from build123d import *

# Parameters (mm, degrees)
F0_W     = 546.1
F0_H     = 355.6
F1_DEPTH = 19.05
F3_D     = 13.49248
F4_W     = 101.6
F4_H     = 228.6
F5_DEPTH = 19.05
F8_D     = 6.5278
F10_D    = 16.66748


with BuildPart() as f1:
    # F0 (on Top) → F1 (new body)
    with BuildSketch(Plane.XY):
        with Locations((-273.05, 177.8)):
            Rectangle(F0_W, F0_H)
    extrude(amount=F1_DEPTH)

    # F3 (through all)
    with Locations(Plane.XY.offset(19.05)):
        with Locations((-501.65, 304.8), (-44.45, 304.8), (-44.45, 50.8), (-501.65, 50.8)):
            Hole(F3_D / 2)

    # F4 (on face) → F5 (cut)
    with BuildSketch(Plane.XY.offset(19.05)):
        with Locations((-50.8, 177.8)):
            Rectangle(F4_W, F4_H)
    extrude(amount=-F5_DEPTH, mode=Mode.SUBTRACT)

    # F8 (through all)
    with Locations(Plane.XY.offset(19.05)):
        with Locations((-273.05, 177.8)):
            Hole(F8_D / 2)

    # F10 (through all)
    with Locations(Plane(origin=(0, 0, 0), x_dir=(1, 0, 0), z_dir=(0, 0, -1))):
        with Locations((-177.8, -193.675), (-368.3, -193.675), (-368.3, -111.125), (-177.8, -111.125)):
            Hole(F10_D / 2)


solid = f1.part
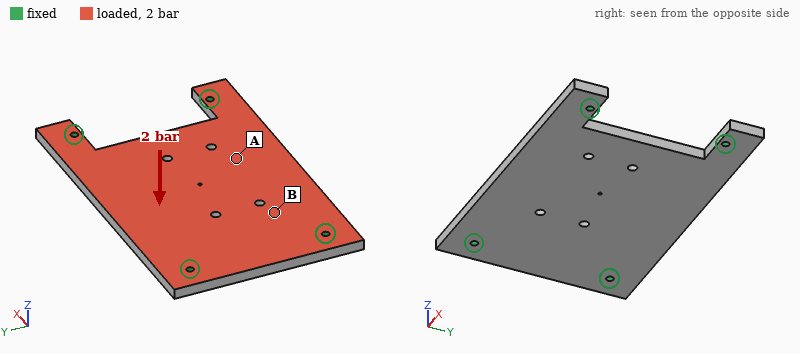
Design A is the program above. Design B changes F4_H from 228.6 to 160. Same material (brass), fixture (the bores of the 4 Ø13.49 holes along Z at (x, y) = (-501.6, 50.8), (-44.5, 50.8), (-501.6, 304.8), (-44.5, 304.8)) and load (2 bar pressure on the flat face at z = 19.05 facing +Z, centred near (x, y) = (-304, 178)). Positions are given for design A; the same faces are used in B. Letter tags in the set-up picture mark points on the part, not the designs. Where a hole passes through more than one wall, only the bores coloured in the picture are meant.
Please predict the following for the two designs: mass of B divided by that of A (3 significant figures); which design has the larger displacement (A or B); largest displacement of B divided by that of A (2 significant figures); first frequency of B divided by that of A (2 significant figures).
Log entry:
1.04
A
0.90
1.1
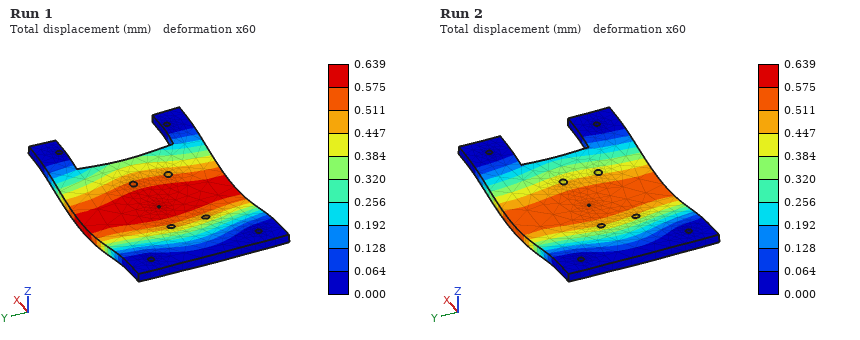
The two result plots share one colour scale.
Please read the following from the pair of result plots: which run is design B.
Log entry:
Run 2
